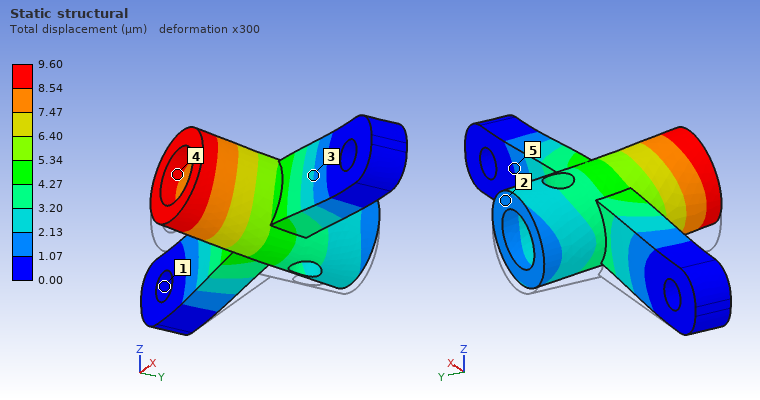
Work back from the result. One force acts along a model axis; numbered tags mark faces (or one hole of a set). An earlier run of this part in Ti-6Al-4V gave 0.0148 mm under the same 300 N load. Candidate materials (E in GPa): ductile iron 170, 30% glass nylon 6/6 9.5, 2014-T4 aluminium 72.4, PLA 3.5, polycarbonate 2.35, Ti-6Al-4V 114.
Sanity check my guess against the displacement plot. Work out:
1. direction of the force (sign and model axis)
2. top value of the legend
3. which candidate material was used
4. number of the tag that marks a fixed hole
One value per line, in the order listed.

+Z
9.60 µm
ductile iron
1
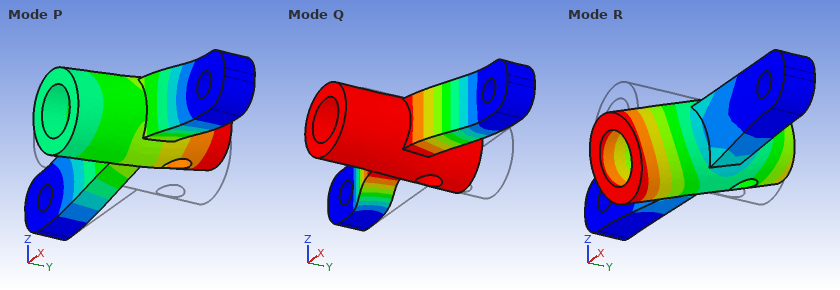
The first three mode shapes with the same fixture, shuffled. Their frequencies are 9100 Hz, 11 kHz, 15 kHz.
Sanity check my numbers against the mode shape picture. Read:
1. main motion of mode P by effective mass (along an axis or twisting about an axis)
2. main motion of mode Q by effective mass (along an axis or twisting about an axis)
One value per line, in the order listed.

along Z
along Y
